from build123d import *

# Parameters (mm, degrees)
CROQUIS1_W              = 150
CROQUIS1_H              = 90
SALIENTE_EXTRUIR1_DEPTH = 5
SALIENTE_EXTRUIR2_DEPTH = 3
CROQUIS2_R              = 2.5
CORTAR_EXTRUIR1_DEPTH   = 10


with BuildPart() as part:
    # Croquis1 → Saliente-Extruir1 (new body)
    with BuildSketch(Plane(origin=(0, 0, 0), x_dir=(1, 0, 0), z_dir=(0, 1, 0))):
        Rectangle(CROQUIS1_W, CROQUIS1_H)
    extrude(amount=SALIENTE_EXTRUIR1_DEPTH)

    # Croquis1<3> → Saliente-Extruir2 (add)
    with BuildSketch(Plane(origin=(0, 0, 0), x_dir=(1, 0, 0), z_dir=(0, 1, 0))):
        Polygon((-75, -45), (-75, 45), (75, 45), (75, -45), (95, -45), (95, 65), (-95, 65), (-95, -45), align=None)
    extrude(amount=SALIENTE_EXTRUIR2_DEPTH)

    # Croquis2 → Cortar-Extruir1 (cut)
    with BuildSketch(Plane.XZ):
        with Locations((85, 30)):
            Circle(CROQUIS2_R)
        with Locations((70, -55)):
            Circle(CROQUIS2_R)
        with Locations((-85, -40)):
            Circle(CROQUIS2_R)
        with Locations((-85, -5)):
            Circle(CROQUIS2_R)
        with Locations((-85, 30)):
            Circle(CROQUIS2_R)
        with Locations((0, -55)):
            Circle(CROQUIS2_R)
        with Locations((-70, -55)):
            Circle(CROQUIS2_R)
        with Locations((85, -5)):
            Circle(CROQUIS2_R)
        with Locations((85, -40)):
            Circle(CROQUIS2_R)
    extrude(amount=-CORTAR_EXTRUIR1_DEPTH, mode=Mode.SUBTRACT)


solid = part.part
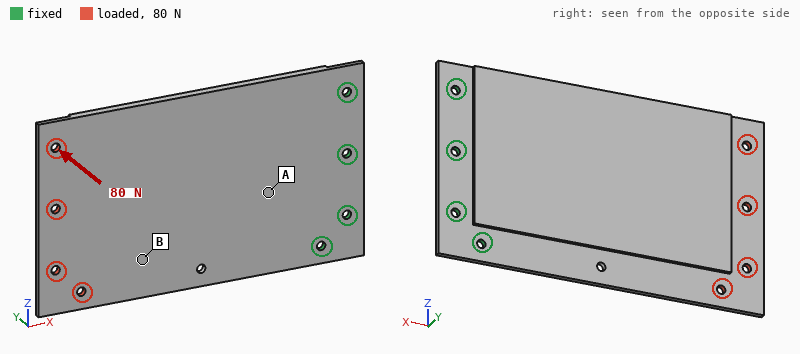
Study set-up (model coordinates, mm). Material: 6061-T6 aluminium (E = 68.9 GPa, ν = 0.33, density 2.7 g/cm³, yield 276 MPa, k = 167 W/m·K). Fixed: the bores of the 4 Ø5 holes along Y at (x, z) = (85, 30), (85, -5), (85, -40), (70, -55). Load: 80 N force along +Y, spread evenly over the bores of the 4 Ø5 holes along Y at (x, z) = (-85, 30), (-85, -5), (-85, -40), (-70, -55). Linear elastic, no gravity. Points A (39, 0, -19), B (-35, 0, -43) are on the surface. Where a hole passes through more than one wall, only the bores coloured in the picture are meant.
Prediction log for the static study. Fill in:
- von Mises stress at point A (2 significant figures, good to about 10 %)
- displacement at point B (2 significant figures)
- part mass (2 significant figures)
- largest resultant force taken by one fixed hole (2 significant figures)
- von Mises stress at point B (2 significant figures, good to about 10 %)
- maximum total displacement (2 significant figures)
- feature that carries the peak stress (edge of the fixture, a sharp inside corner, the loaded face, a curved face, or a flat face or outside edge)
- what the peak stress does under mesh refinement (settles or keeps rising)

24 MPa
1.4 mm
240 g
430 N
8.6 MPa
2.6 mm
edge of the fixture
keeps rising
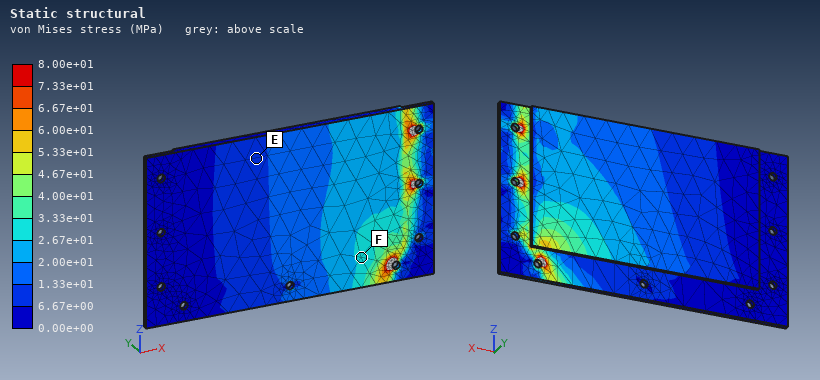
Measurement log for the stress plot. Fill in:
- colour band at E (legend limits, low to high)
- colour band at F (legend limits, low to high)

6.67e+00 to 1.33e+01 MPa
2.67e+01 to 3.33e+01 MPa
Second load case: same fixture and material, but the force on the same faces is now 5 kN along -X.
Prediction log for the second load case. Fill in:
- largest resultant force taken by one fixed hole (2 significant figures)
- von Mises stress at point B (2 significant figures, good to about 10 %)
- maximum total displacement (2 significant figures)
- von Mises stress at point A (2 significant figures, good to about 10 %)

1.4 kN
23 MPa
0.78 mm
18 MPa
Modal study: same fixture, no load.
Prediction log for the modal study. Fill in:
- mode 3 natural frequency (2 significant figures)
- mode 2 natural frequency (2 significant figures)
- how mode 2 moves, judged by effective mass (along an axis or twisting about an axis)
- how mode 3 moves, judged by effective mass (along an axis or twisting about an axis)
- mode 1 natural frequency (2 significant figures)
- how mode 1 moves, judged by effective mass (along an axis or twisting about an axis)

760 Hz
460 Hz
twisting about X
along Y
110 Hz
along Y
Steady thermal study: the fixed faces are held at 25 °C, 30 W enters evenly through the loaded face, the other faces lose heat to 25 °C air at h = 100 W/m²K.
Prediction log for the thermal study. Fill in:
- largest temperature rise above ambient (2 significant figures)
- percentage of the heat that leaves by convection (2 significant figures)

23 K
91 %
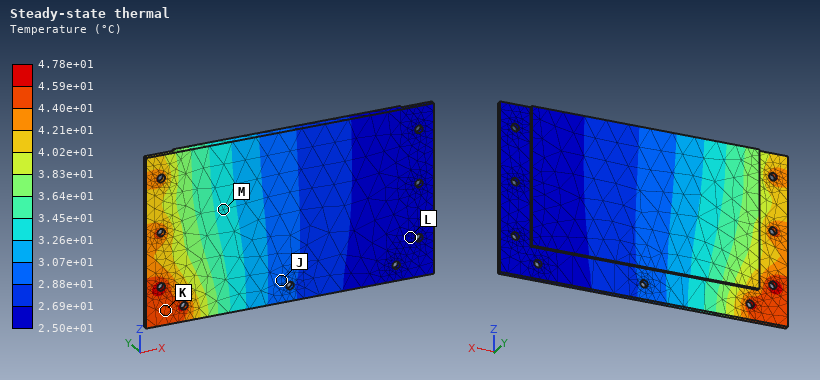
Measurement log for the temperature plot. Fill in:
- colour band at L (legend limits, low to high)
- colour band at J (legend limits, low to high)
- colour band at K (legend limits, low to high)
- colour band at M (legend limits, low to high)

2.50e+01 to 2.69e+01 °C
2.88e+01 to 3.07e+01 °C
4.40e+01 to 4.59e+01 °C
3.26e+01 to 3.45e+01 °C
